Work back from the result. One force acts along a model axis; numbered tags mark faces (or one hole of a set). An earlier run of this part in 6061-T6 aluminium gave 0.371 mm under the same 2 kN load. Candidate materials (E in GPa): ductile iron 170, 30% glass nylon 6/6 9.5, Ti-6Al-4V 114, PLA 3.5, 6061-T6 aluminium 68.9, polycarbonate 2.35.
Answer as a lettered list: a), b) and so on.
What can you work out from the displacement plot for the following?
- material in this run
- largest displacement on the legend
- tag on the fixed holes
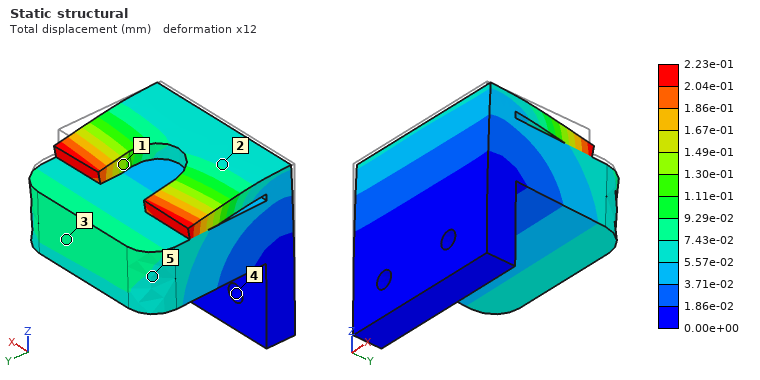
a) Ti-6Al-4V
b) 2.23e-01 mm
c) 4
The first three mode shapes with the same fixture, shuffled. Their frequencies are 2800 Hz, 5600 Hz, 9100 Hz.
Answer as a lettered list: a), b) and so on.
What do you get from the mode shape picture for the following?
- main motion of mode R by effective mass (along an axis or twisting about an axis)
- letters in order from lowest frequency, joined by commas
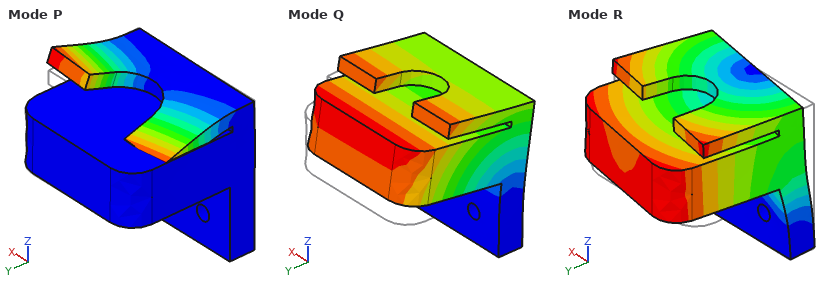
a) along X
b) Q, R, P
